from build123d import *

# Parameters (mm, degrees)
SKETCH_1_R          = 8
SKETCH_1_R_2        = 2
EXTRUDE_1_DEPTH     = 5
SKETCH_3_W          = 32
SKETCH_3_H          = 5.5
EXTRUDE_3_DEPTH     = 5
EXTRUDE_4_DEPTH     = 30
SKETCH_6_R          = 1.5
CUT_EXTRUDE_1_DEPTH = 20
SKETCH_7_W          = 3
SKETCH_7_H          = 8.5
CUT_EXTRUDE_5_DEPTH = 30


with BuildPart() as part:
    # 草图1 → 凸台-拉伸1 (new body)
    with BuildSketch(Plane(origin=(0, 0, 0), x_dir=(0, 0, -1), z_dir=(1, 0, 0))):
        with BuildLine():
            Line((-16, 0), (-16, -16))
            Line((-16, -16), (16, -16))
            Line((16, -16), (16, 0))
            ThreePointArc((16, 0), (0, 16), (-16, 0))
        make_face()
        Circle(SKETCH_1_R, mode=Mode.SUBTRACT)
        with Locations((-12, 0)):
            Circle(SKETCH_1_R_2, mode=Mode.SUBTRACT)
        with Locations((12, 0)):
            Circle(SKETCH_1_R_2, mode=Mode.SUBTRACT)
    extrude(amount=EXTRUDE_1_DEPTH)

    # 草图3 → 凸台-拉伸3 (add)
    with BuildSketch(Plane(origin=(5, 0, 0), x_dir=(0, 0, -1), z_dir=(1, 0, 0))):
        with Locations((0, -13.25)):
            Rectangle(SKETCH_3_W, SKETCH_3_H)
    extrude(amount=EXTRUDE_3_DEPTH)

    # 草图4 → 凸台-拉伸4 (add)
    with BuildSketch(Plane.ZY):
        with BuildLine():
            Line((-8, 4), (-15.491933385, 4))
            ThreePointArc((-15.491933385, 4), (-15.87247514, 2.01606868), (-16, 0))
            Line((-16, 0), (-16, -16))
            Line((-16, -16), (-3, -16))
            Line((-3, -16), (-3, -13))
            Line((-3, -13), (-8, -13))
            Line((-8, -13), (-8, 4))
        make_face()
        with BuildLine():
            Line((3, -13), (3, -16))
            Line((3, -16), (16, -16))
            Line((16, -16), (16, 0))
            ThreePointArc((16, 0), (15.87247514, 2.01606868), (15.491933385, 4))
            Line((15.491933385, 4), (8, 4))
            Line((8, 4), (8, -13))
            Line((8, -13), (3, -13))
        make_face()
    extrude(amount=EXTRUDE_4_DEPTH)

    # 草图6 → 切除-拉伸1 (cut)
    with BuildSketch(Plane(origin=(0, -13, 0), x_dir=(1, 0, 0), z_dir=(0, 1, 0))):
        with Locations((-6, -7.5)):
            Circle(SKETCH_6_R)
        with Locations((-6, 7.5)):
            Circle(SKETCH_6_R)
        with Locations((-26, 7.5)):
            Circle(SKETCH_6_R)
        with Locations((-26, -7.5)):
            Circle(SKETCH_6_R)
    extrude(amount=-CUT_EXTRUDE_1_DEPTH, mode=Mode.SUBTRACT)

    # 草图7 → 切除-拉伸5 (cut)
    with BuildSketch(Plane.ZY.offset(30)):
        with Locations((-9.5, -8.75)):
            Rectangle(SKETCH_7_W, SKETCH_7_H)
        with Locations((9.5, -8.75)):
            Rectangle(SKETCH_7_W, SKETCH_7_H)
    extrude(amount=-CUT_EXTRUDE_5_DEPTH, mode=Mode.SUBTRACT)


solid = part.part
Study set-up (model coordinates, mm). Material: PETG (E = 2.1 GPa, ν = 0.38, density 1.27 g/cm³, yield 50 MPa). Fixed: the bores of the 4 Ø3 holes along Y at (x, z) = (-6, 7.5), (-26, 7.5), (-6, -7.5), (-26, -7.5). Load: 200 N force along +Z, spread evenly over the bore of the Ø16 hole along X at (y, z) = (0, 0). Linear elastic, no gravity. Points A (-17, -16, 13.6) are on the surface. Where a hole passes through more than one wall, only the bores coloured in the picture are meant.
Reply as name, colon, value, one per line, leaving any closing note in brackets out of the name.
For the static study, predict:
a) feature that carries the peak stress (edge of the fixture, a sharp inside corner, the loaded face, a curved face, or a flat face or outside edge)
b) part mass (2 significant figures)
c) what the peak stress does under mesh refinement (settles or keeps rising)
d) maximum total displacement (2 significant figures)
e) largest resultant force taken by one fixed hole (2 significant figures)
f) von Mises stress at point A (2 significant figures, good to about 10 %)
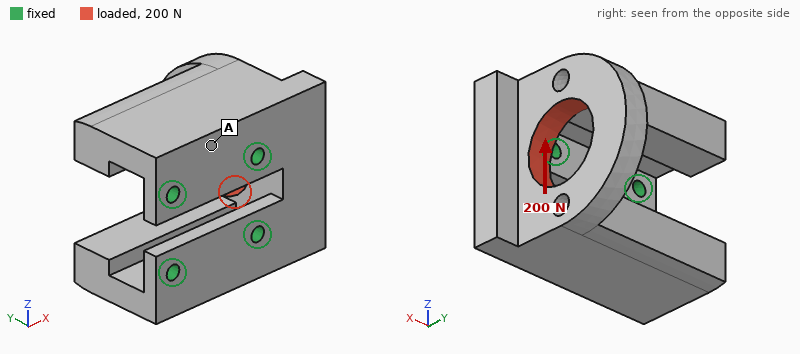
feature that carries the peak stress: edge of the fixture
part mass: 17 g
what the peak stress does under mesh refinement: keeps rising
maximum total displacement: 0.41 mm
largest resultant force taken by one fixed hole: 180 N
von Mises stress at point A: 2.7 MPa
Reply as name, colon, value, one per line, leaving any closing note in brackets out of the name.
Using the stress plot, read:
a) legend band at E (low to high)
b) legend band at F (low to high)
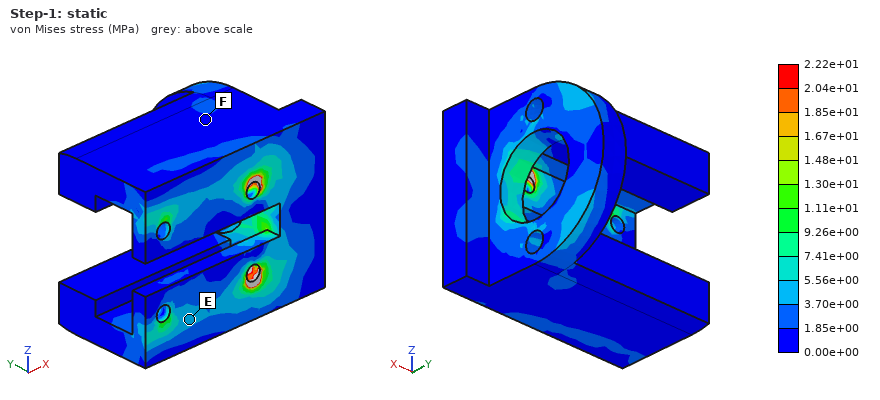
legend band at E: 3.70e+00 to 5.56e+00 MPa
legend band at F: 0.00e+00 to 1.85e+00 MPa
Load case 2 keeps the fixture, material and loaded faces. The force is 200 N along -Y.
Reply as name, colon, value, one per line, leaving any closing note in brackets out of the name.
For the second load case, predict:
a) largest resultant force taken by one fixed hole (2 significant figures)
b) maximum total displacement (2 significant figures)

largest resultant force taken by one fixed hole: 130 N
maximum total displacement: 0.17 mm
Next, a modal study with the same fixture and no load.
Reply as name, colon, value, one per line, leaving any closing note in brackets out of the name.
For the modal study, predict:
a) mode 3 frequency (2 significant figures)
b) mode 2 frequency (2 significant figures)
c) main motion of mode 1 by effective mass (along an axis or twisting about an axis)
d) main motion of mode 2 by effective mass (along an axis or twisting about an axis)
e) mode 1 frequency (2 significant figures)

mode 3 frequency: 2300 Hz
mode 2 frequency: 1800 Hz
main motion of mode 1 by effective mass: along Z
main motion of mode 2 by effective mass: along X
mode 1 frequency: 1300 Hz
